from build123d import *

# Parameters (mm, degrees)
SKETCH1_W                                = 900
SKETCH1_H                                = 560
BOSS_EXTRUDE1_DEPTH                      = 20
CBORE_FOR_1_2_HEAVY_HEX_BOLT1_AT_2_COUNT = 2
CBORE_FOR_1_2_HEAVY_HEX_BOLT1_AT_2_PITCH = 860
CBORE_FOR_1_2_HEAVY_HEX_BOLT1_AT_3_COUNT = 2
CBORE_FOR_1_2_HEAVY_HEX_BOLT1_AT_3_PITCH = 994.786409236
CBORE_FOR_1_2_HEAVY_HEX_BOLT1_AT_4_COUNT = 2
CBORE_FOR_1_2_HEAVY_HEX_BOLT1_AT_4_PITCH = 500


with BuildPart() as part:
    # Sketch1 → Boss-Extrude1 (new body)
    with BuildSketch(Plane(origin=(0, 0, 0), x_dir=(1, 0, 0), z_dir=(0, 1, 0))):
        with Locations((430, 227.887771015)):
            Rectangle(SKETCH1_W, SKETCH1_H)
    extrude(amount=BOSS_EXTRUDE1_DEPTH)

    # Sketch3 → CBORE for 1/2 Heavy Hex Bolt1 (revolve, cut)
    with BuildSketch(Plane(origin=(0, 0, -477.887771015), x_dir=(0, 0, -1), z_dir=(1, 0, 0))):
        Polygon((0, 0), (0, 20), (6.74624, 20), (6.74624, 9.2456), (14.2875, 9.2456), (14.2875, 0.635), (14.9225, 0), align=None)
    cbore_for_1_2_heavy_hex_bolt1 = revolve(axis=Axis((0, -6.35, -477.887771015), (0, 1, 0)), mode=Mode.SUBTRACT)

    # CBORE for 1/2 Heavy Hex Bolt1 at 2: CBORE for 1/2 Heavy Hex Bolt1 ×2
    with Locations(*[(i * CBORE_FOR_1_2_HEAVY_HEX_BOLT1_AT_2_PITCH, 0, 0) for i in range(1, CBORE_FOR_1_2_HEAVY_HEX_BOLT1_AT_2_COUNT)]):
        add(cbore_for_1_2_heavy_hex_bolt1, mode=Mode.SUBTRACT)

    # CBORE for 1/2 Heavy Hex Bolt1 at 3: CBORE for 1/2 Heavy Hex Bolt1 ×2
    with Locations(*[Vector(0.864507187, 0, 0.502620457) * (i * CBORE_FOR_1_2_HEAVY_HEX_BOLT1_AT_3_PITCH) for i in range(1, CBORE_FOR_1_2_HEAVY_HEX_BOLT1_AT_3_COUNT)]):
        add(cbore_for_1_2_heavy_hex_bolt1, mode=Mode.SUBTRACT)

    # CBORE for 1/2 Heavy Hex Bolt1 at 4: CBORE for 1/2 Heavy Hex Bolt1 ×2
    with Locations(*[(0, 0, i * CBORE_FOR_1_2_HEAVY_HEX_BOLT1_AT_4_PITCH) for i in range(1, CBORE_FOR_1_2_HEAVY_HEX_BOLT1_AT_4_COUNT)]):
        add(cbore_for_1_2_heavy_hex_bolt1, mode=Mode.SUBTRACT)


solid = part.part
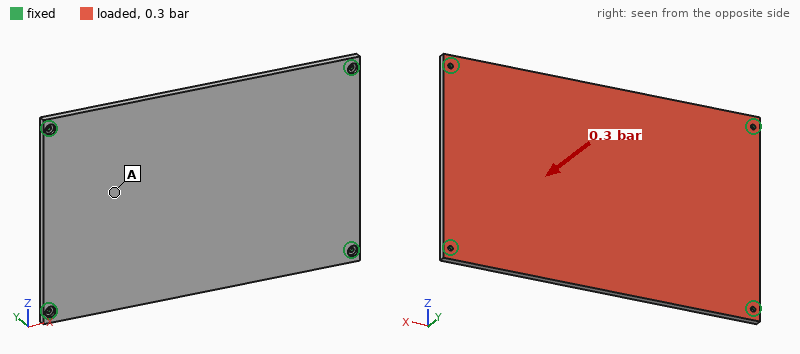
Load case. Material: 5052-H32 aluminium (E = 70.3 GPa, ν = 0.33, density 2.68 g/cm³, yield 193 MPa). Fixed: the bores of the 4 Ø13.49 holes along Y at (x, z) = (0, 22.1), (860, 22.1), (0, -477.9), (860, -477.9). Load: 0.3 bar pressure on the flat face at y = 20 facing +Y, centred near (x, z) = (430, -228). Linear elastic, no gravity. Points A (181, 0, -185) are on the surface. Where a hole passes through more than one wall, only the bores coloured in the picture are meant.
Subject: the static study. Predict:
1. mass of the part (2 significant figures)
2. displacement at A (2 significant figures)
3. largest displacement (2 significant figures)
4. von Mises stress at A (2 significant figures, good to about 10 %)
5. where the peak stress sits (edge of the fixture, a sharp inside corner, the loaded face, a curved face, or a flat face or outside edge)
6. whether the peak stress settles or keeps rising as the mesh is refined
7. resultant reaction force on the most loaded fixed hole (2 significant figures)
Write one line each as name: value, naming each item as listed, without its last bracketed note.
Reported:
mass of the part: 27 kg
displacement at A: 1.3 mm
largest displacement: 2.1 mm
von Mises stress at A: 11 MPa
where the peak stress sits: edge of the fixture
whether the peak stress settles or keeps rising as the mesh is refined: keeps rising
resultant reaction force on the most loaded fixed hole: 11 kN
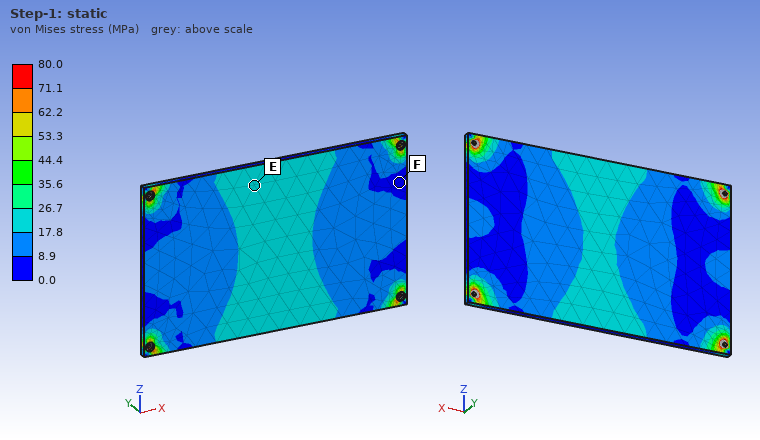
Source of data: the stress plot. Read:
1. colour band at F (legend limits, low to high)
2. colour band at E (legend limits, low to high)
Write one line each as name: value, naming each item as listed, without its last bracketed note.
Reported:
colour band at F: 0.0 to 8.9 MPa
colour band at E: 17.8 to 26.7 MPa
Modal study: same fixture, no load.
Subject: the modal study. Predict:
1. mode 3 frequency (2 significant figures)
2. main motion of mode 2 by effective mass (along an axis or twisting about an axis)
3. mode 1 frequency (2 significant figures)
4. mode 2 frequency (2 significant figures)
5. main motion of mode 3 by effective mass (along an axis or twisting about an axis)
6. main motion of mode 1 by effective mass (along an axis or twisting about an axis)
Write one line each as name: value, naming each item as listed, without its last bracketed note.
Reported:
mode 3 frequency: 260 Hz
main motion of mode 2 by effective mass: twisting about X
mode 1 frequency: 93 Hz
mode 2 frequency: 180 Hz
main motion of mode 3 by effective mass: twisting about Z
main motion of mode 1 by effective mass: along Y
